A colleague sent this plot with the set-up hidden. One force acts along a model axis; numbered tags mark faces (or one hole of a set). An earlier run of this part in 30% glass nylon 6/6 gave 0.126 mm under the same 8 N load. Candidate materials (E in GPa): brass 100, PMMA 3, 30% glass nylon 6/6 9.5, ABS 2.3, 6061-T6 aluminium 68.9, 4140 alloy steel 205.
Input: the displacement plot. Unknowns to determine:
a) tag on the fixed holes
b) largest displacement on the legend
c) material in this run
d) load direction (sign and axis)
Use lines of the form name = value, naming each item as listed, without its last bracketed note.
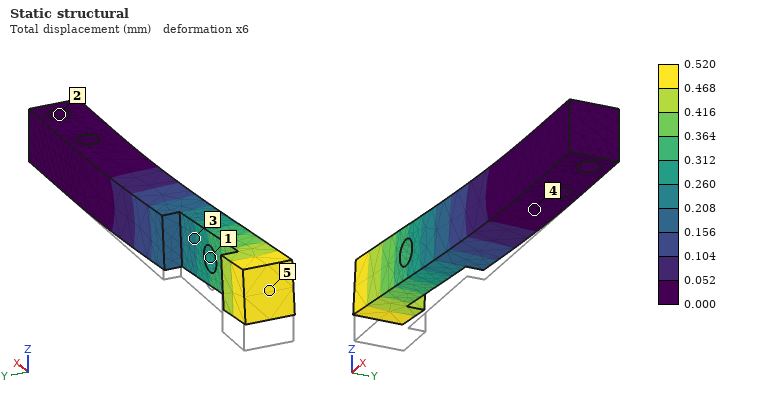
tag on the fixed holes = 2
largest displacement on the legend = 0.520 mm
material in this run = ABS
load direction = +Z
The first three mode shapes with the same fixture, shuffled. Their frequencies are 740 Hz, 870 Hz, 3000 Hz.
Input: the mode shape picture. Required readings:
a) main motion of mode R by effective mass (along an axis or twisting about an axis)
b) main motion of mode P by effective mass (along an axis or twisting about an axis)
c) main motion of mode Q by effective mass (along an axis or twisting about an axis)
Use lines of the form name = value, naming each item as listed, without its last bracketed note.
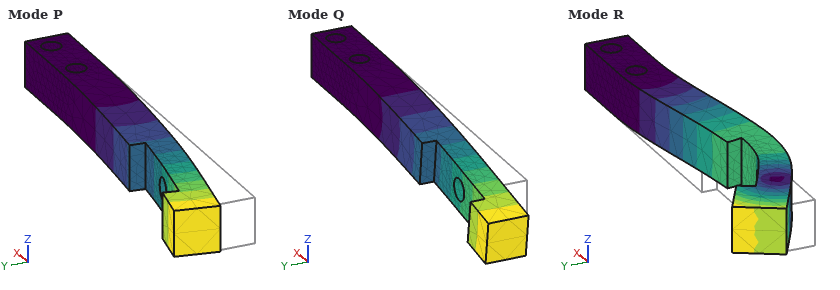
main motion of mode R by effective mass = along Y
main motion of mode P by effective mass = along Y
main motion of mode Q by effective mass = along Z
